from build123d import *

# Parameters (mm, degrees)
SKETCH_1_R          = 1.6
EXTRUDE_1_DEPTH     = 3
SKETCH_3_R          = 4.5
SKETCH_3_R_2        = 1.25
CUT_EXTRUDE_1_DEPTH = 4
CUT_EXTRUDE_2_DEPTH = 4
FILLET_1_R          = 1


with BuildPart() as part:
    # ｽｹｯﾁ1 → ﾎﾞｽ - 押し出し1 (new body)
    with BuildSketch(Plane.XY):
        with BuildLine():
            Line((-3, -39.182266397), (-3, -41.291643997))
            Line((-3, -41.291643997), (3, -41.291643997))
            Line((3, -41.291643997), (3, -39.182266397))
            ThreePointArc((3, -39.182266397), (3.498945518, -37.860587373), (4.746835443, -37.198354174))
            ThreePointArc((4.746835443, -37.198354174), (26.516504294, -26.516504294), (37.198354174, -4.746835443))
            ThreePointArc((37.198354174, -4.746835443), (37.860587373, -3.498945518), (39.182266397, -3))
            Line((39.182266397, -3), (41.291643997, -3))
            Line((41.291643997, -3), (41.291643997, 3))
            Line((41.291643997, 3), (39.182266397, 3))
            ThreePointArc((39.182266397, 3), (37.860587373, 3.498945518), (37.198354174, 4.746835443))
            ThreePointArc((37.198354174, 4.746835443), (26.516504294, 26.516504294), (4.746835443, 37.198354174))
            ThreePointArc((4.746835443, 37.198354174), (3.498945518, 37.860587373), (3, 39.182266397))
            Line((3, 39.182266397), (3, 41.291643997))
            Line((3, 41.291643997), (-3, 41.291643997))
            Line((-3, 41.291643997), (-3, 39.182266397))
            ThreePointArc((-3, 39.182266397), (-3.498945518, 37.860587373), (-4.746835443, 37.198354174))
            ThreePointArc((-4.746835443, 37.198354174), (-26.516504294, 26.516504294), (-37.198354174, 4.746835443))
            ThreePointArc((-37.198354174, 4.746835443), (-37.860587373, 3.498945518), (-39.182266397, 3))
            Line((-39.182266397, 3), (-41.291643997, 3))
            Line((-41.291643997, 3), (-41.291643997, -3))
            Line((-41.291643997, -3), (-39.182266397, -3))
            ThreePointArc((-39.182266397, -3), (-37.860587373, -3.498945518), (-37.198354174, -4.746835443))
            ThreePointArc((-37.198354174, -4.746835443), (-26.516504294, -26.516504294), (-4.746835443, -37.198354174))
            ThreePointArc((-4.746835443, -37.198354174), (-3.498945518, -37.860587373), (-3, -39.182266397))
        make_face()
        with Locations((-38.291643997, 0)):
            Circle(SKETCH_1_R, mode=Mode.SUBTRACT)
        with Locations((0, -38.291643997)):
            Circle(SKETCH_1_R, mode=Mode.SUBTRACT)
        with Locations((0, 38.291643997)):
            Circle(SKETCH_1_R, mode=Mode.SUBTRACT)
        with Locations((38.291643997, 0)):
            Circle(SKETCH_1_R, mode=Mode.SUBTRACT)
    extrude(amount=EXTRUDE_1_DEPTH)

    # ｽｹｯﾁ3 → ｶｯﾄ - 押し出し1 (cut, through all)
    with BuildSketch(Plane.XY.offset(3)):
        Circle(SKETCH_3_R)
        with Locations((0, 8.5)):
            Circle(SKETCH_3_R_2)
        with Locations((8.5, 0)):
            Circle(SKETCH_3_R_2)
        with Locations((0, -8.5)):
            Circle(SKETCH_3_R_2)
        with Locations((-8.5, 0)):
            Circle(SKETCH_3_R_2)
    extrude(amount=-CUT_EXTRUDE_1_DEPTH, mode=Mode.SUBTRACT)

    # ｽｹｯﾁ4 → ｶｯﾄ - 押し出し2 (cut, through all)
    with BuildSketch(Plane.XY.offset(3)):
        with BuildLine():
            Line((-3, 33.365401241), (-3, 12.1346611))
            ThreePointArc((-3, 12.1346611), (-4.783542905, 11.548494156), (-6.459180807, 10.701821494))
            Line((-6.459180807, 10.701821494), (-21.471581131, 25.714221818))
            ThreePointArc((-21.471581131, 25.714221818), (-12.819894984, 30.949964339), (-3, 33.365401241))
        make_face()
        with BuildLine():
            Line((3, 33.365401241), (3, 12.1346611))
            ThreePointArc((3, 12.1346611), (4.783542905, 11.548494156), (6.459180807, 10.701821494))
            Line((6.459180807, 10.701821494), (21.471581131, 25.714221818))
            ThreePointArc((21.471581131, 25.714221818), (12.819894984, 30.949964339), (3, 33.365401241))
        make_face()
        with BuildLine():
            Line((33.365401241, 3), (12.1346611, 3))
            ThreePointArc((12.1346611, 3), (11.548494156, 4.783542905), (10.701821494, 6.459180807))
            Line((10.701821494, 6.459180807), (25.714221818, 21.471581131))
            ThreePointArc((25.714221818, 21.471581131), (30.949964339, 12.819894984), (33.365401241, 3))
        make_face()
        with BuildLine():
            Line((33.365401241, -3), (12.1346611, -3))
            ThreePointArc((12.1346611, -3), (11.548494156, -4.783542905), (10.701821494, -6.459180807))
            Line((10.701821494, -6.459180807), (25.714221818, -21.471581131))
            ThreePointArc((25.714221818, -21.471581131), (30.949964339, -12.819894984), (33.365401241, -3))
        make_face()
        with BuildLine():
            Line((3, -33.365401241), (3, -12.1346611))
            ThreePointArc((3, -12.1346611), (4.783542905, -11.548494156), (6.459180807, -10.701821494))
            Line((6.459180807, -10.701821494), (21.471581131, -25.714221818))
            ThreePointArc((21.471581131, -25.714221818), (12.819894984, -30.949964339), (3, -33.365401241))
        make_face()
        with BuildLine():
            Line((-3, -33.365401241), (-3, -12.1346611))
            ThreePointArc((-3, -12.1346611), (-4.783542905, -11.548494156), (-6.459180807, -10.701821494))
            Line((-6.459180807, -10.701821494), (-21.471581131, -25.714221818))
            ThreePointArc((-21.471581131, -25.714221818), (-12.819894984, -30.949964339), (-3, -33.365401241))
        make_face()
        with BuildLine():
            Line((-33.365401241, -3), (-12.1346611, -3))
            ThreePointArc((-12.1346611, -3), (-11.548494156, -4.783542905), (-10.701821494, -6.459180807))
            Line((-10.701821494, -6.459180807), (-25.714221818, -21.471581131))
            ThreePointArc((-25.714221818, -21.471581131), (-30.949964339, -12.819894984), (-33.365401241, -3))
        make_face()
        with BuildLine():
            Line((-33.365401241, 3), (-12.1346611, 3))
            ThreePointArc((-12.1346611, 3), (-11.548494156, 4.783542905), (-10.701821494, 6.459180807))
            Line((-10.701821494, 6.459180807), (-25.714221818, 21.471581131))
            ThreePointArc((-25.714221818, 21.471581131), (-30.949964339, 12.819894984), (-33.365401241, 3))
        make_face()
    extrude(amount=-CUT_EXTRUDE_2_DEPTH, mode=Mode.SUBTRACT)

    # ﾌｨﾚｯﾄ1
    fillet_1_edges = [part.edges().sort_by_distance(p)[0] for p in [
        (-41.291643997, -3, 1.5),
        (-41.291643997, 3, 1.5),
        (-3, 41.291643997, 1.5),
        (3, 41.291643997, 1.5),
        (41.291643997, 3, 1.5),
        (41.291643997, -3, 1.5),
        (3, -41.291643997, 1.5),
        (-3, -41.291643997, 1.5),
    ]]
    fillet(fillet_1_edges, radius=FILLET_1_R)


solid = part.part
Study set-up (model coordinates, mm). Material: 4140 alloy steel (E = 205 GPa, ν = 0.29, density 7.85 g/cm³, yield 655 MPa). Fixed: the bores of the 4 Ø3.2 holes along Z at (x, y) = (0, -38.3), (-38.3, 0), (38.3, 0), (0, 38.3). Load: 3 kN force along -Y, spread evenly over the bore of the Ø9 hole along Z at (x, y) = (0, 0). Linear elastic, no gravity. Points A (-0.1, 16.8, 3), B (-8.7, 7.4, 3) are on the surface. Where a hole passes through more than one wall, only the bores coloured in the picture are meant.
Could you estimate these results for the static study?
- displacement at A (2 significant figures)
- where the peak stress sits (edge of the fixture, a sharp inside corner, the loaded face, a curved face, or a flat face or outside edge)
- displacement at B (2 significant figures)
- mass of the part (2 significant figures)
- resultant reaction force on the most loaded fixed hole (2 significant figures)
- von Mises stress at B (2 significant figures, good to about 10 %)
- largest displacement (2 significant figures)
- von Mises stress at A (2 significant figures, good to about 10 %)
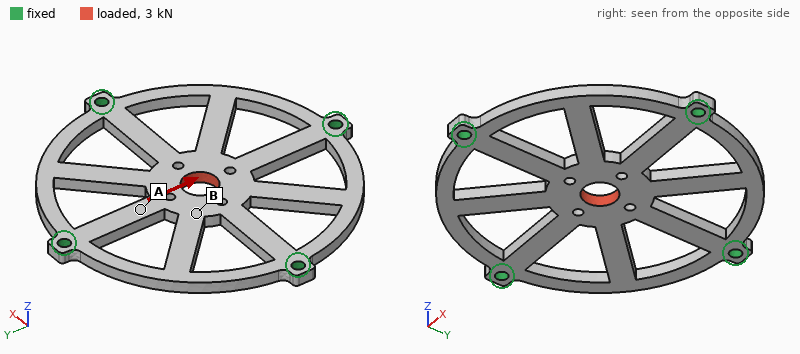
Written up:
6.8 µm
a curved face
9.8 µm
56 g
1.1 kN
16 MPa
11 µm
67 MPa
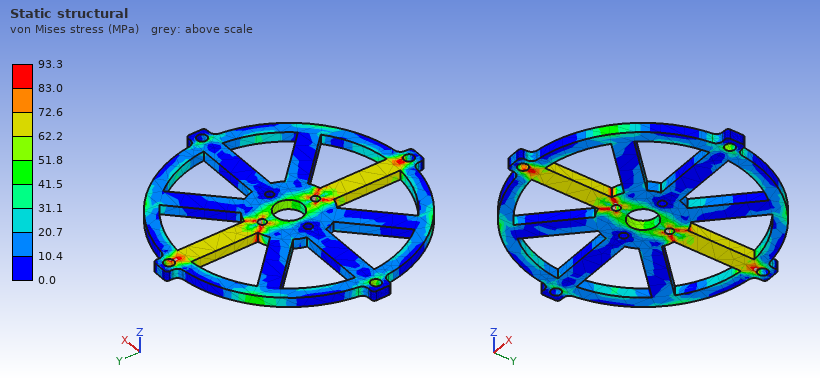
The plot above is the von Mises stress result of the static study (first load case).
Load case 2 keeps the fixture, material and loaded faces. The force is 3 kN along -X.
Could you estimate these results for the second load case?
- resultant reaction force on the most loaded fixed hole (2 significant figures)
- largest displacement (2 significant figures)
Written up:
1.1 kN
11 µm
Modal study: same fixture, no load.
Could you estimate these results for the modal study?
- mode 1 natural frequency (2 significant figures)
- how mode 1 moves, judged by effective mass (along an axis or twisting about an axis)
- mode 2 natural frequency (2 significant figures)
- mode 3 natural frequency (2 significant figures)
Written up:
2900 Hz
along Z
4300 Hz
4400 Hz
